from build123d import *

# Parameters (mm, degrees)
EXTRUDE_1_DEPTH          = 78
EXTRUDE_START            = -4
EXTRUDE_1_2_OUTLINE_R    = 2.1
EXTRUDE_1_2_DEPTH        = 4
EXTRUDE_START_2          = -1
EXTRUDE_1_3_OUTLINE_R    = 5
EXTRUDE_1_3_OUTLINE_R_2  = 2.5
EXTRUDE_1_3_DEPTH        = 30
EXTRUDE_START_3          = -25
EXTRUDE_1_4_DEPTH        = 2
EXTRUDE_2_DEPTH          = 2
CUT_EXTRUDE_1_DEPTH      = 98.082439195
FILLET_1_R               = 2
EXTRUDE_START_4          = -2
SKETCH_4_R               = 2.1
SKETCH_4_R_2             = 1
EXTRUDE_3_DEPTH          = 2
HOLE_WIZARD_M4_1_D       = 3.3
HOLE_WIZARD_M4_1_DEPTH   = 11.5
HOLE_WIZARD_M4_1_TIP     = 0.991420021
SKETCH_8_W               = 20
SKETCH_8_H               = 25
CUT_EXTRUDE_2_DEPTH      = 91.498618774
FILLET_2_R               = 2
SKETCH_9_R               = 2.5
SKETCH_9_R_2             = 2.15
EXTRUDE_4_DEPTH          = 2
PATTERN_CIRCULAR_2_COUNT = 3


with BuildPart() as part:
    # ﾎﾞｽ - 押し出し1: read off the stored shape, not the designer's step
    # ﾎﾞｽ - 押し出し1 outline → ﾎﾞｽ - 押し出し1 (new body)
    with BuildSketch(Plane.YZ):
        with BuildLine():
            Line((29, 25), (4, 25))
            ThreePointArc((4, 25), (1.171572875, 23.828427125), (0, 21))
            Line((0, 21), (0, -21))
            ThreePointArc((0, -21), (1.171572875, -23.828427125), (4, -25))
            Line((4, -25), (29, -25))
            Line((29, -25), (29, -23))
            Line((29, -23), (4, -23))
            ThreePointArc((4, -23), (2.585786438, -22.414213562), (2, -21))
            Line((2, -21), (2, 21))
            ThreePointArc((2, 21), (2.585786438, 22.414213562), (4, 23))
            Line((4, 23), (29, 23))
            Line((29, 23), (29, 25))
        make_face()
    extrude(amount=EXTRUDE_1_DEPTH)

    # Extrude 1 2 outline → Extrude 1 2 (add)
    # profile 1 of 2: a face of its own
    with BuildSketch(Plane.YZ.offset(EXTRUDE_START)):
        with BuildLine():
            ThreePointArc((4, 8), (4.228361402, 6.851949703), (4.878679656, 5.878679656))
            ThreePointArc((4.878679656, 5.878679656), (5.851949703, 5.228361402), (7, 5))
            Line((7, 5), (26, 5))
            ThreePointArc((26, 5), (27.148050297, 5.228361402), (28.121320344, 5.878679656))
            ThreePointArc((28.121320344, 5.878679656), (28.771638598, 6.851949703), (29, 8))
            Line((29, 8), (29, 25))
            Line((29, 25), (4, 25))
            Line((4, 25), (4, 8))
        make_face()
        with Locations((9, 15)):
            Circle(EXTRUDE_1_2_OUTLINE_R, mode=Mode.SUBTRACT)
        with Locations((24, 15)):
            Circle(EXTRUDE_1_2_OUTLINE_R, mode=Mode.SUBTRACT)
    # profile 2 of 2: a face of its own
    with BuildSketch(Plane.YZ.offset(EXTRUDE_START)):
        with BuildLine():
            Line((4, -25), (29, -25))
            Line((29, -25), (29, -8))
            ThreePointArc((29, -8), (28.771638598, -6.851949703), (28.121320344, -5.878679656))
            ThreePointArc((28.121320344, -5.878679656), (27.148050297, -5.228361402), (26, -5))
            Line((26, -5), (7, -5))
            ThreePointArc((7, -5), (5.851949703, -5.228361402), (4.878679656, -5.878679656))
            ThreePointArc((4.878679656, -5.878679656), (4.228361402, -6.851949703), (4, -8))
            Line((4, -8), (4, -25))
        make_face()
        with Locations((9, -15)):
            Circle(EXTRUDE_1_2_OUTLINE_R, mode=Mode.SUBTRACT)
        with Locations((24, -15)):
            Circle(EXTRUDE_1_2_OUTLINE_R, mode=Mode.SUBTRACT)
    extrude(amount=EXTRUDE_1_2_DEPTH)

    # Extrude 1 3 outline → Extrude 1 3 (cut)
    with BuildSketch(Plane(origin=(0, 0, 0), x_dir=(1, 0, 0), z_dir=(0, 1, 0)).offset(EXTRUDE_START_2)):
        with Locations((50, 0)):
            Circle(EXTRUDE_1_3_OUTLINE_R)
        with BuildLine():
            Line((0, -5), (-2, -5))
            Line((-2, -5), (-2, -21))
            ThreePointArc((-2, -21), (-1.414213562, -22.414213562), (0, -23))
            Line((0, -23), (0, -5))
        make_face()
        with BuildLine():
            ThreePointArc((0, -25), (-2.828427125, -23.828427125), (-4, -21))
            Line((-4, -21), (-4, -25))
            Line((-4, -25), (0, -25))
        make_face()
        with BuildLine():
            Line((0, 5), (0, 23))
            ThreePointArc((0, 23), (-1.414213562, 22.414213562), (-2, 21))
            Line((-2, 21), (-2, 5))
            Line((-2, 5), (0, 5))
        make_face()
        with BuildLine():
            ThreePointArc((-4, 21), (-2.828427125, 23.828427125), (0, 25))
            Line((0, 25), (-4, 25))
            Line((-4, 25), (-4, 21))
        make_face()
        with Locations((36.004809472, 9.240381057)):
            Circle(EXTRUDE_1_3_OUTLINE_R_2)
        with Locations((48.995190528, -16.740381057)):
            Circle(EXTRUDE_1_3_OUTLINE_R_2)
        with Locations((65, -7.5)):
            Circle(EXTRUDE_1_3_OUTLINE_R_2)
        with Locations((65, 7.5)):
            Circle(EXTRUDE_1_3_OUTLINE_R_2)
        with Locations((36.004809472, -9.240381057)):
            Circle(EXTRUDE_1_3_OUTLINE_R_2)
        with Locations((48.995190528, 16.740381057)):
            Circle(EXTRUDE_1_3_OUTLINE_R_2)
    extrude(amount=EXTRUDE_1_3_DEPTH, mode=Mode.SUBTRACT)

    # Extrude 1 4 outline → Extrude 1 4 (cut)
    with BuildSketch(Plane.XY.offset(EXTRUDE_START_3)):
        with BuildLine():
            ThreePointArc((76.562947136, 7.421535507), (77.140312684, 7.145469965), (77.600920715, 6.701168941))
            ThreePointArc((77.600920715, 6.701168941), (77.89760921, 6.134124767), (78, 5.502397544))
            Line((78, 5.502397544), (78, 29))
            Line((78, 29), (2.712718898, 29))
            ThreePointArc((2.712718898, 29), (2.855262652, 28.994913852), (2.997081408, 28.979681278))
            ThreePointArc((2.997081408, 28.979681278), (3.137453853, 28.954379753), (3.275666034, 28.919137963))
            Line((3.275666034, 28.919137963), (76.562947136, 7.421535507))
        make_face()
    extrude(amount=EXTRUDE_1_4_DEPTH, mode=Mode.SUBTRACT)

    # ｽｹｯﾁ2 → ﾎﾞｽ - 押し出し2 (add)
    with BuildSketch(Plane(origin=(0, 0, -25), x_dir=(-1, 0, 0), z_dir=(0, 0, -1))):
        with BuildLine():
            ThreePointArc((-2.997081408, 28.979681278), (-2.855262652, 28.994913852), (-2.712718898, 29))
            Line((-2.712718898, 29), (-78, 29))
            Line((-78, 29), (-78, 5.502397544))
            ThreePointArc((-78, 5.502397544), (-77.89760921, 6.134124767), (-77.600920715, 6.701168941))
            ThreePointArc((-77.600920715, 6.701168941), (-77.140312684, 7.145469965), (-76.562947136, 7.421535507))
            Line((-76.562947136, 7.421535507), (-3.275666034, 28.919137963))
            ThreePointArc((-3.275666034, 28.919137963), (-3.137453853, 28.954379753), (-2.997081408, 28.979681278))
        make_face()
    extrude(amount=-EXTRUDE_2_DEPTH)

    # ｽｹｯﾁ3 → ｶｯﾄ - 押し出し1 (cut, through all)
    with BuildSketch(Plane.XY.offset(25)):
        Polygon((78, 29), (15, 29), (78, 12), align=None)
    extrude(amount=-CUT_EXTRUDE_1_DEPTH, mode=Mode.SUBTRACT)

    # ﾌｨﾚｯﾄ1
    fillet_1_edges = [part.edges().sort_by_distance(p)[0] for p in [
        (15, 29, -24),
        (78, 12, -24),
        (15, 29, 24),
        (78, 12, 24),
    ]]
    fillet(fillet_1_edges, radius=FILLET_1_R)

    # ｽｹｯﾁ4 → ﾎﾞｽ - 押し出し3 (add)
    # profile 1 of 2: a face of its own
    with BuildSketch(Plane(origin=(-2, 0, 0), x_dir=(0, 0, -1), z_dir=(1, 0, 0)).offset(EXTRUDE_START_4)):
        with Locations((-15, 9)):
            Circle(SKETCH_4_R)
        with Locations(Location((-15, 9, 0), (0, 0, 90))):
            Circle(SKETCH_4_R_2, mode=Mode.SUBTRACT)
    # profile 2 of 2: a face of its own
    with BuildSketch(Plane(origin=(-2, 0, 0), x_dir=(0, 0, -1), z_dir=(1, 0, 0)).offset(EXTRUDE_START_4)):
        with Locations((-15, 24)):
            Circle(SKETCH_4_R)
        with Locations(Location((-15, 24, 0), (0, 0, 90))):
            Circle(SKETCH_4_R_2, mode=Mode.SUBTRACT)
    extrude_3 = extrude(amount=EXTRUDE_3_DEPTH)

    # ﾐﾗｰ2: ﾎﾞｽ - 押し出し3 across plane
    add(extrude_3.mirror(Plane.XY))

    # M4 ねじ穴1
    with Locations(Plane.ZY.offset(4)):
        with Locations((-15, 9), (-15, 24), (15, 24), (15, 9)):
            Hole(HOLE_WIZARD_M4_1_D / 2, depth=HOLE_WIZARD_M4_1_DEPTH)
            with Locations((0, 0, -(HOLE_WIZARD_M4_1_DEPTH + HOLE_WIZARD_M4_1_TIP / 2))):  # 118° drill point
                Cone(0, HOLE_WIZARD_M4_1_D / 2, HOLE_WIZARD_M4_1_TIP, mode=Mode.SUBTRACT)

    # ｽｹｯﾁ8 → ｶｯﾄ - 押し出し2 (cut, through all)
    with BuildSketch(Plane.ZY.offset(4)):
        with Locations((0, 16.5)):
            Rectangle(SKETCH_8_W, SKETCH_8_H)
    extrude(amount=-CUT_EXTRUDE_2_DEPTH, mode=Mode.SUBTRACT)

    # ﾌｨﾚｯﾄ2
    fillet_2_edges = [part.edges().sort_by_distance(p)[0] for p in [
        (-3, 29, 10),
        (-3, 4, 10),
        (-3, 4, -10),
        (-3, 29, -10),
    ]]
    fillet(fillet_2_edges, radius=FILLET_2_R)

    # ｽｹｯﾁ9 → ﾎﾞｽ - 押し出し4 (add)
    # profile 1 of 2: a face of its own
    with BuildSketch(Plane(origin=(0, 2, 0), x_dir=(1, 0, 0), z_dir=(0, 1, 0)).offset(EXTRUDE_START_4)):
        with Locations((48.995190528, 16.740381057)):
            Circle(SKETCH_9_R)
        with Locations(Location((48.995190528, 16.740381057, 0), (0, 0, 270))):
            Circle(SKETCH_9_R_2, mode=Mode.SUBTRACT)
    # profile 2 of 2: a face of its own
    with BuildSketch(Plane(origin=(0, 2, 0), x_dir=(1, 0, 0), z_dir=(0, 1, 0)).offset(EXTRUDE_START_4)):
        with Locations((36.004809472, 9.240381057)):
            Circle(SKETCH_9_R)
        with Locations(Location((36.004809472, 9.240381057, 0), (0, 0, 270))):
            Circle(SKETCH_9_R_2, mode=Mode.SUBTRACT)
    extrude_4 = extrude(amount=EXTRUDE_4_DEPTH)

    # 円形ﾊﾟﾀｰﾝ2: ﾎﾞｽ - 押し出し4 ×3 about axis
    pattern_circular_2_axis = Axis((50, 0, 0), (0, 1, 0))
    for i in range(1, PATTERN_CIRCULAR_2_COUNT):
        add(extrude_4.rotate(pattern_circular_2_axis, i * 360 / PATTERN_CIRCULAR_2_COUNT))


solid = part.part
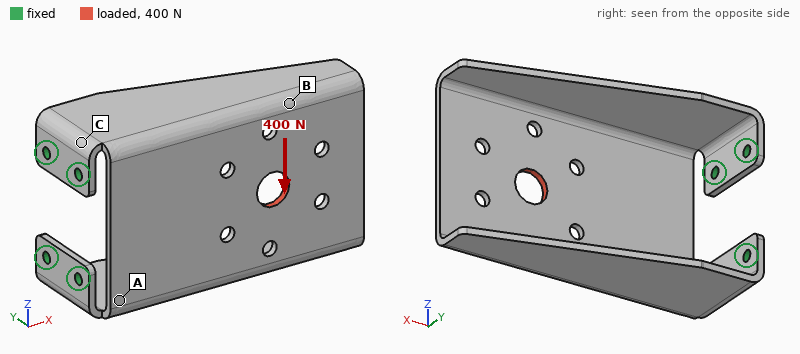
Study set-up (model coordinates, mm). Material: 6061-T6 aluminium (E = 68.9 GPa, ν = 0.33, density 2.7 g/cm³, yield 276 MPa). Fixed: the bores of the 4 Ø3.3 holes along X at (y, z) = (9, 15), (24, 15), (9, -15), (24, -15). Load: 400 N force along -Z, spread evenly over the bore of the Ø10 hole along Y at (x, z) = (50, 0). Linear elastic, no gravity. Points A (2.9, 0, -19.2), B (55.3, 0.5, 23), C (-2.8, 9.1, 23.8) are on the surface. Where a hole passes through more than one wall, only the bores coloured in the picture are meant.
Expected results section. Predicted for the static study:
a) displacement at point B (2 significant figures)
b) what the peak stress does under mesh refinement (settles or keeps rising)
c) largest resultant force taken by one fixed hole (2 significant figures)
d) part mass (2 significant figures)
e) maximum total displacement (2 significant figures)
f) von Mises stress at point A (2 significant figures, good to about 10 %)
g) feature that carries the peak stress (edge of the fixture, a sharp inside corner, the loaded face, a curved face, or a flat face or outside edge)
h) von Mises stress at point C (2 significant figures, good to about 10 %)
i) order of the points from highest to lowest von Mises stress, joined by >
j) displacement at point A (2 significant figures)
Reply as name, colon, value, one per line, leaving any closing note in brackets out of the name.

displacement at point B: 0.64 mm
what the peak stress does under mesh refinement: keeps rising
largest resultant force taken by one fixed hole: 510 N
part mass: 40 g
maximum total displacement: 0.99 mm
von Mises stress at point A: 53 MPa
feature that carries the peak stress: edge of the fixture
von Mises stress at point C: 88 MPa
order of the points from highest to lowest von Mises stress, joined by >: C > A > B
displacement at point A: 0.21 mm
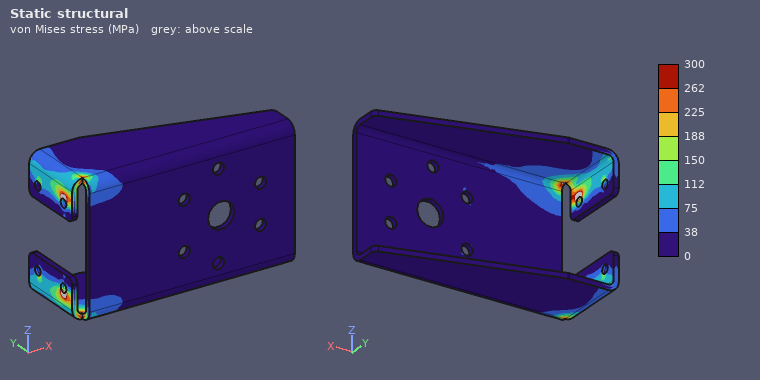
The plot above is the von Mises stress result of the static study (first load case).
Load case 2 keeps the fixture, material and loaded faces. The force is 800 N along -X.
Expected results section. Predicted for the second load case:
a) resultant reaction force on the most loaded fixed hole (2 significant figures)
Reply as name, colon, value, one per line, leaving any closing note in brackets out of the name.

resultant reaction force on the most loaded fixed hole: 600 N
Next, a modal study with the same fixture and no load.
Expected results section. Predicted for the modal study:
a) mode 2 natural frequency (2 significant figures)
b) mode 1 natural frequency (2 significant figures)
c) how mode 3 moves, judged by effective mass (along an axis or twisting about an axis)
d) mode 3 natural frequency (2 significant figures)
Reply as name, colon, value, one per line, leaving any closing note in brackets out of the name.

mode 2 natural frequency: 720 Hz
mode 1 natural frequency: 710 Hz
how mode 3 moves, judged by effective mass: along Z
mode 3 natural frequency: 1800 Hz
